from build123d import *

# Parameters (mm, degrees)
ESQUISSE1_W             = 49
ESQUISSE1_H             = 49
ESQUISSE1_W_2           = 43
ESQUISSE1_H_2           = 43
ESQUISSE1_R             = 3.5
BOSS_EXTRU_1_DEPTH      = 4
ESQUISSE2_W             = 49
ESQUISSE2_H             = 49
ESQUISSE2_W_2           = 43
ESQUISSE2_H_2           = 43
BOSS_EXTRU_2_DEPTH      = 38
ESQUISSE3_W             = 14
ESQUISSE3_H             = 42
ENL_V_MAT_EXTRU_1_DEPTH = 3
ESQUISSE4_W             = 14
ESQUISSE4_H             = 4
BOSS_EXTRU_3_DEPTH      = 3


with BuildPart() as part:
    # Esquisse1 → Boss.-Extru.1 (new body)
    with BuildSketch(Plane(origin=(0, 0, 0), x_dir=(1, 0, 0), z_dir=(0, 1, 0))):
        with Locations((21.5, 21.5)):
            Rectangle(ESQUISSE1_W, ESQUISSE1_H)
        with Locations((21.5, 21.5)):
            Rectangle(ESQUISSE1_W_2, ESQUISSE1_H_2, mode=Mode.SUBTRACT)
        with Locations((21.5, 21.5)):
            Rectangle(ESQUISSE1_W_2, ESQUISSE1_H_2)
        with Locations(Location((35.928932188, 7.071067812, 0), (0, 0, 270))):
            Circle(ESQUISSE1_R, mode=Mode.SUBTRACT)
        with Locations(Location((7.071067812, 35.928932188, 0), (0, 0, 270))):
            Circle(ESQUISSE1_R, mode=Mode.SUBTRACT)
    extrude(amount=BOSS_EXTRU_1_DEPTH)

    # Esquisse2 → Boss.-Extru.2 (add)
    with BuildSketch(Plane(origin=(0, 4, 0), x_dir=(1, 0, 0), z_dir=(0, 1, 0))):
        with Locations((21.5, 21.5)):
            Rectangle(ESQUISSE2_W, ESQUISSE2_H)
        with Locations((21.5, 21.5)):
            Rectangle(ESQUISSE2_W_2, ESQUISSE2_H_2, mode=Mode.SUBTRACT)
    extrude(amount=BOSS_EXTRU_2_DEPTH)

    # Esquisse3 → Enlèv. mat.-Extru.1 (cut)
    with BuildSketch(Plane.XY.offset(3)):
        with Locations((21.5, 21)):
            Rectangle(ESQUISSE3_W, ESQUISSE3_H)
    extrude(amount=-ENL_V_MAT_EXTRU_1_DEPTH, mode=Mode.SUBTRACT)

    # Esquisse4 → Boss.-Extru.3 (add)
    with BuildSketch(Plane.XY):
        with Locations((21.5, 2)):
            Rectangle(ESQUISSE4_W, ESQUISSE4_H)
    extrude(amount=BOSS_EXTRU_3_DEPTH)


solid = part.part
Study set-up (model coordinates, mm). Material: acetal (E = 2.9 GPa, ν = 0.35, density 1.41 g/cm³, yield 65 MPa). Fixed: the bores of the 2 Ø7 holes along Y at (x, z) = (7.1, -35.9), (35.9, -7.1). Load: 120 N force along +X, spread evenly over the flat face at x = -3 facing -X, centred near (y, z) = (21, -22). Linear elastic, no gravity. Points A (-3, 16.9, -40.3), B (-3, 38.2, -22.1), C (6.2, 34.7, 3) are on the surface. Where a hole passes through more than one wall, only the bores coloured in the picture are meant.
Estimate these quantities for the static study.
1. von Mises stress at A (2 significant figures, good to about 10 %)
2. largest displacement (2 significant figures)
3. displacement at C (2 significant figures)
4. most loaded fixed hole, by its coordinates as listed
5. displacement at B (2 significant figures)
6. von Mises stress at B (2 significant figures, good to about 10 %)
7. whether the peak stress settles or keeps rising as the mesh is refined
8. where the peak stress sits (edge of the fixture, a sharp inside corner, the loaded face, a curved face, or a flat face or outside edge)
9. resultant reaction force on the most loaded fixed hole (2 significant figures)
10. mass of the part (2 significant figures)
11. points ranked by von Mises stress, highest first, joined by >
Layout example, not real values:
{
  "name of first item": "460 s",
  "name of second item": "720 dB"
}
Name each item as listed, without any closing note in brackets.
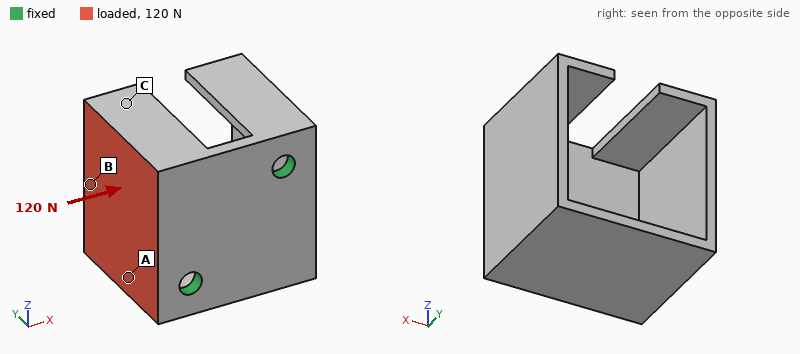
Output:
{
  "von Mises stress at A": "2.6 MPa",
  "largest displacement": "0.78 mm",
  "displacement at C": "0.57 mm",
  "most loaded fixed hole, by its coordinates as listed": "(7.1, -35.9)",
  "displacement at B": "0.61 mm",
  "von Mises stress at B": "5.4 MPa",
  "whether the peak stress settles or keeps rising as the mesh is refined": "keeps rising",
  "where the peak stress sits": "edge of the fixture",
  "resultant reaction force on the most loaded fixed hole": "79 N",
  "mass of the part": "40 g",
  "points ranked by von Mises stress, highest first, joined by >": "B > A > C"
}
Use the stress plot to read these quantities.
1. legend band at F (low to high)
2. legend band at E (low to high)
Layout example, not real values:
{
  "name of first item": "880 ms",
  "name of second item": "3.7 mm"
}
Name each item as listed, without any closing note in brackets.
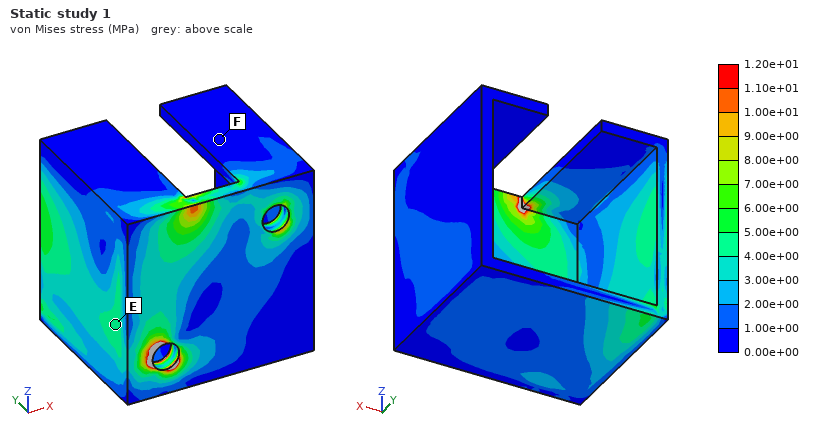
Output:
{
  "legend band at F": "0.00e+00 to 1.00e+00 MPa",
  "legend band at E": "4.00e+00 to 5.00e+00 MPa"
}
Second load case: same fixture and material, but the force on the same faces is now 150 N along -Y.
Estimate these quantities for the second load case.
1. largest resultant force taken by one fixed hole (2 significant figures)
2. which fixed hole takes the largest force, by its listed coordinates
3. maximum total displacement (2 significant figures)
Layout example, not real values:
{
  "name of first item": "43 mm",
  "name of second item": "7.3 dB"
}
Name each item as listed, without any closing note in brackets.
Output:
{
  "largest resultant force taken by one fixed hole": "140 N",
  "which fixed hole takes the largest force, by its listed coordinates": "(7.1, -35.9)",
  "maximum total displacement": "0.85 mm"
}
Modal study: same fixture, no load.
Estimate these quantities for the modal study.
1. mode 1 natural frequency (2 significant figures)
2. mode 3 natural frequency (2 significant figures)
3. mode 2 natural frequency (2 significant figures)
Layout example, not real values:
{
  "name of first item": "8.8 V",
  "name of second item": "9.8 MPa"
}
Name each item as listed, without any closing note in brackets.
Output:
{
  "mode 1 natural frequency": "530 Hz",
  "mode 3 natural frequency": "940 Hz",
  "mode 2 natural frequency": "650 Hz"
}
